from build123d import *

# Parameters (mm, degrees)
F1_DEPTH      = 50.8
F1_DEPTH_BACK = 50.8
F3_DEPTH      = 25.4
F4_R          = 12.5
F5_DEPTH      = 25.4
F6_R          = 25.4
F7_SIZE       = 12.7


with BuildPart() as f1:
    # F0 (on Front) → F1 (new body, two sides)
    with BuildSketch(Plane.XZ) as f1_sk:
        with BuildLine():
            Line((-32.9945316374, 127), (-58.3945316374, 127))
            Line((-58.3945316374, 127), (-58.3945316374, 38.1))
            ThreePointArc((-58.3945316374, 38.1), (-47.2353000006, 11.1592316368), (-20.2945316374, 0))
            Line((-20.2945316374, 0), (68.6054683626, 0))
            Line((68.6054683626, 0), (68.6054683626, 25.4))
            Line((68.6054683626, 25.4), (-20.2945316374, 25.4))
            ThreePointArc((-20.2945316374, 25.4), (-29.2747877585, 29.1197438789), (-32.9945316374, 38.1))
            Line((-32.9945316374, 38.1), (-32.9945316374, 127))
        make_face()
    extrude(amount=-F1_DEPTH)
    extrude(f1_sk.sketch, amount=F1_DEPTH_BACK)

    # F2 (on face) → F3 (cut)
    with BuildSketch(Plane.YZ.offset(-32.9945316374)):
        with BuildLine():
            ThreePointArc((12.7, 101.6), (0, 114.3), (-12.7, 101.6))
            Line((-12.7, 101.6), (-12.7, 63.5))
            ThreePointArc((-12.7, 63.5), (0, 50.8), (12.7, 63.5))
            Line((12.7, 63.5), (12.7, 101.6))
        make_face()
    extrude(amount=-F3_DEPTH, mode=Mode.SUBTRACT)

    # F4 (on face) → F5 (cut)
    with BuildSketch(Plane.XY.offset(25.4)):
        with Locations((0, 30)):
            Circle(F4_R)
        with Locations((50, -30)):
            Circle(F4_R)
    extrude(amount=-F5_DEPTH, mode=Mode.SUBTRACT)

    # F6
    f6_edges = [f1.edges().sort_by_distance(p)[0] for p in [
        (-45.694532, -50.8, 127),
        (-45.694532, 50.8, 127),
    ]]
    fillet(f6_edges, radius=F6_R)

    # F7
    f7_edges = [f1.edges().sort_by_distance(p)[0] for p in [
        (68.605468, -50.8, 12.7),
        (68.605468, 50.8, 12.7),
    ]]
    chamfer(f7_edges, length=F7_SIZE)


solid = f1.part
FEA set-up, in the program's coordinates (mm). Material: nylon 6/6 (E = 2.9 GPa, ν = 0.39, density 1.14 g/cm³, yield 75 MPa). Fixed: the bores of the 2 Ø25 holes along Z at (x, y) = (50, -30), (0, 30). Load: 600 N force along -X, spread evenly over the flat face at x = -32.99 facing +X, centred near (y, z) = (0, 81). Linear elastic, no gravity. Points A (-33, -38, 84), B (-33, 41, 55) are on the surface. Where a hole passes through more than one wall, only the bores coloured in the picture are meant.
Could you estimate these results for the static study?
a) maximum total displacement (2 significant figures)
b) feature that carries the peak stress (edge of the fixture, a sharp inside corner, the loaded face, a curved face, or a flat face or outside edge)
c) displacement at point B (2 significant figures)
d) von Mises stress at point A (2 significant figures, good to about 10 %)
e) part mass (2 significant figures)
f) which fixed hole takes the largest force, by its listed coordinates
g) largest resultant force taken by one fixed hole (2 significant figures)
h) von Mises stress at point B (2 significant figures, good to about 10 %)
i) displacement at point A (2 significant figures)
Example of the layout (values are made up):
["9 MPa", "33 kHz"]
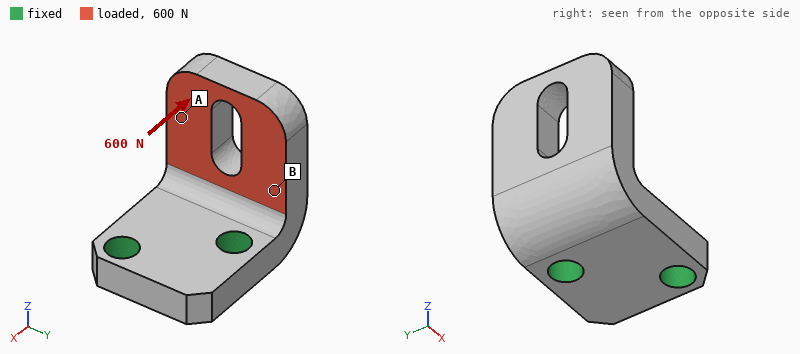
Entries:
["0.79 mm", "a flat face or outside edge", "0.20 mm", "0.70 MPa", "560 g", "(0, 30)", "410 N", "1.8 MPa", "0.43 mm"]
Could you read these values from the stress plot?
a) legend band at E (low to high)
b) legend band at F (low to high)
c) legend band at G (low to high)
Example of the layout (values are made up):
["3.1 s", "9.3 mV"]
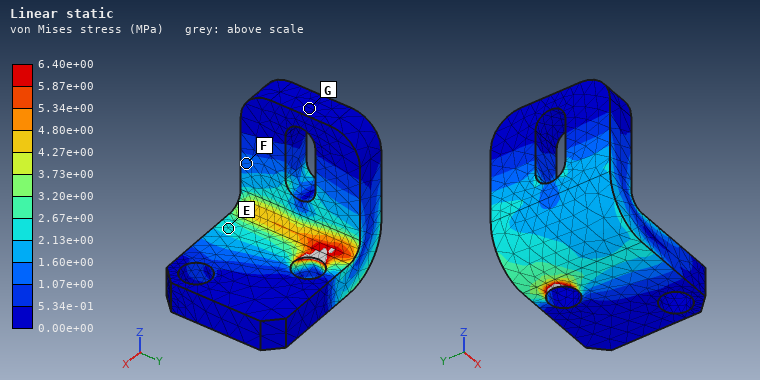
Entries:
["2.13e+00 to 2.67e+00 MPa", "1.07e+00 to 1.60e+00 MPa", "0.00e+00 to 5.34e-01 MPa"]
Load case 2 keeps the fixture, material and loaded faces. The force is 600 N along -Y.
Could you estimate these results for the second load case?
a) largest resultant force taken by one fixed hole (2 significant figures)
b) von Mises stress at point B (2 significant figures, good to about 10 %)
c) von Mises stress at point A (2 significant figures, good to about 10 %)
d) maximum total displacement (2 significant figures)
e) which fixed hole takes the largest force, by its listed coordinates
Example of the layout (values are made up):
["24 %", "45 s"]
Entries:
["650 N", "1.5 MPa", "0.95 MPa", "0.44 mm", "(0, 30)"]
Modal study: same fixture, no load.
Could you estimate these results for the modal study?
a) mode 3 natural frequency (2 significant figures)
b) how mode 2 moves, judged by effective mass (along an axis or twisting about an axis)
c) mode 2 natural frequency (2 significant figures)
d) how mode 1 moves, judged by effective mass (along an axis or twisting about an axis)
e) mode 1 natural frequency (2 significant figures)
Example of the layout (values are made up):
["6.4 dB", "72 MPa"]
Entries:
["1000 Hz", "along Y", "500 Hz", "along X", "350 Hz"]
